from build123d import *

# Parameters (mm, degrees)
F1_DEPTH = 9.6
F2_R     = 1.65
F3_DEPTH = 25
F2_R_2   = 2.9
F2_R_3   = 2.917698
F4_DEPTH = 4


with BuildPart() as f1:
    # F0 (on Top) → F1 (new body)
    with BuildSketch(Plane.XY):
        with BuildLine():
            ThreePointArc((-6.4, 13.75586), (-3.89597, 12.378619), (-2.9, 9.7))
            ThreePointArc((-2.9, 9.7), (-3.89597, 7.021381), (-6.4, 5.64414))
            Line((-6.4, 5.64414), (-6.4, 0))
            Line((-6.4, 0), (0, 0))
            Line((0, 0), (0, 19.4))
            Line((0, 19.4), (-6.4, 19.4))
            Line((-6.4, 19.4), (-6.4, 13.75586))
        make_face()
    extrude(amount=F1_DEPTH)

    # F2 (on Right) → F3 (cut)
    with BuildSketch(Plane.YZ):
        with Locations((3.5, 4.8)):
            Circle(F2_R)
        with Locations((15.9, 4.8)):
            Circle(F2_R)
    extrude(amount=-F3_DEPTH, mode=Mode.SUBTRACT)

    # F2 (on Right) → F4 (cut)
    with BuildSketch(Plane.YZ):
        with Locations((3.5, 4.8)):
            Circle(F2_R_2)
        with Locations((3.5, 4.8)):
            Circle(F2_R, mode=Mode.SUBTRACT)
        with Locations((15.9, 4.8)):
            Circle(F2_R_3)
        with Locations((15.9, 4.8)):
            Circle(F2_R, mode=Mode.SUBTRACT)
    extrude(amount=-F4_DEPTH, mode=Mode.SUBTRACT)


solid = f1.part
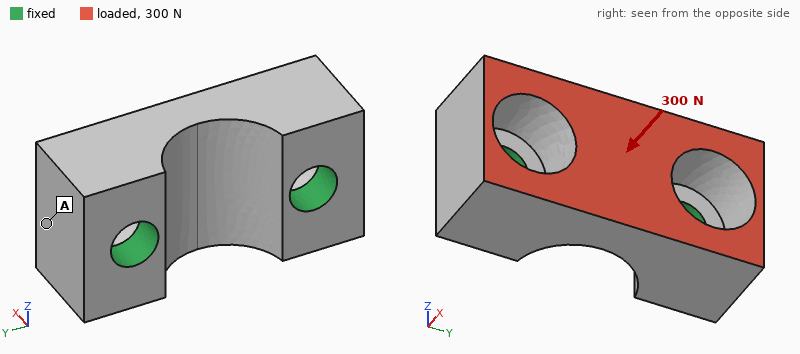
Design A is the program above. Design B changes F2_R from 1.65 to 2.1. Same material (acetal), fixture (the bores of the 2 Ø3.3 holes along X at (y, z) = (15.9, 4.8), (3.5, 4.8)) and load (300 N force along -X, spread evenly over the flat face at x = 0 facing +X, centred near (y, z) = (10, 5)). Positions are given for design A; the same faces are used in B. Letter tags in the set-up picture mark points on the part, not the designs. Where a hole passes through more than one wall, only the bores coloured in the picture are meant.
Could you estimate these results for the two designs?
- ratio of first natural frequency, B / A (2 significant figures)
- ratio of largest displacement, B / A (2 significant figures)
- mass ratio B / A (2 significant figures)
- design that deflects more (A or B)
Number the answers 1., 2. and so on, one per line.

1. 1.2
2. 0.80
3. 0.97
4. A
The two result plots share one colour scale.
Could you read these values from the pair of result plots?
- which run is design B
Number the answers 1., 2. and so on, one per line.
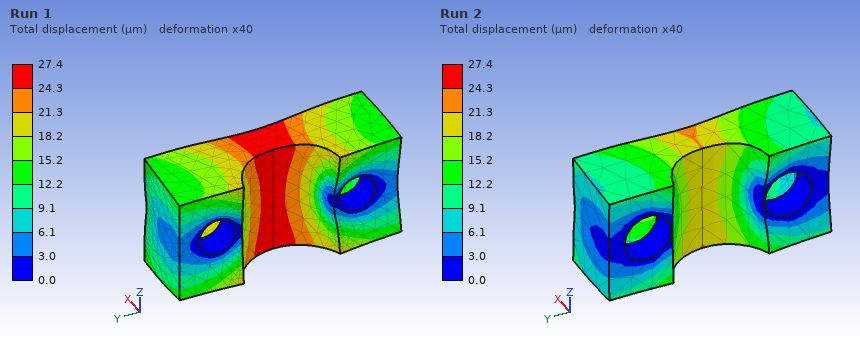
1. Run 2
